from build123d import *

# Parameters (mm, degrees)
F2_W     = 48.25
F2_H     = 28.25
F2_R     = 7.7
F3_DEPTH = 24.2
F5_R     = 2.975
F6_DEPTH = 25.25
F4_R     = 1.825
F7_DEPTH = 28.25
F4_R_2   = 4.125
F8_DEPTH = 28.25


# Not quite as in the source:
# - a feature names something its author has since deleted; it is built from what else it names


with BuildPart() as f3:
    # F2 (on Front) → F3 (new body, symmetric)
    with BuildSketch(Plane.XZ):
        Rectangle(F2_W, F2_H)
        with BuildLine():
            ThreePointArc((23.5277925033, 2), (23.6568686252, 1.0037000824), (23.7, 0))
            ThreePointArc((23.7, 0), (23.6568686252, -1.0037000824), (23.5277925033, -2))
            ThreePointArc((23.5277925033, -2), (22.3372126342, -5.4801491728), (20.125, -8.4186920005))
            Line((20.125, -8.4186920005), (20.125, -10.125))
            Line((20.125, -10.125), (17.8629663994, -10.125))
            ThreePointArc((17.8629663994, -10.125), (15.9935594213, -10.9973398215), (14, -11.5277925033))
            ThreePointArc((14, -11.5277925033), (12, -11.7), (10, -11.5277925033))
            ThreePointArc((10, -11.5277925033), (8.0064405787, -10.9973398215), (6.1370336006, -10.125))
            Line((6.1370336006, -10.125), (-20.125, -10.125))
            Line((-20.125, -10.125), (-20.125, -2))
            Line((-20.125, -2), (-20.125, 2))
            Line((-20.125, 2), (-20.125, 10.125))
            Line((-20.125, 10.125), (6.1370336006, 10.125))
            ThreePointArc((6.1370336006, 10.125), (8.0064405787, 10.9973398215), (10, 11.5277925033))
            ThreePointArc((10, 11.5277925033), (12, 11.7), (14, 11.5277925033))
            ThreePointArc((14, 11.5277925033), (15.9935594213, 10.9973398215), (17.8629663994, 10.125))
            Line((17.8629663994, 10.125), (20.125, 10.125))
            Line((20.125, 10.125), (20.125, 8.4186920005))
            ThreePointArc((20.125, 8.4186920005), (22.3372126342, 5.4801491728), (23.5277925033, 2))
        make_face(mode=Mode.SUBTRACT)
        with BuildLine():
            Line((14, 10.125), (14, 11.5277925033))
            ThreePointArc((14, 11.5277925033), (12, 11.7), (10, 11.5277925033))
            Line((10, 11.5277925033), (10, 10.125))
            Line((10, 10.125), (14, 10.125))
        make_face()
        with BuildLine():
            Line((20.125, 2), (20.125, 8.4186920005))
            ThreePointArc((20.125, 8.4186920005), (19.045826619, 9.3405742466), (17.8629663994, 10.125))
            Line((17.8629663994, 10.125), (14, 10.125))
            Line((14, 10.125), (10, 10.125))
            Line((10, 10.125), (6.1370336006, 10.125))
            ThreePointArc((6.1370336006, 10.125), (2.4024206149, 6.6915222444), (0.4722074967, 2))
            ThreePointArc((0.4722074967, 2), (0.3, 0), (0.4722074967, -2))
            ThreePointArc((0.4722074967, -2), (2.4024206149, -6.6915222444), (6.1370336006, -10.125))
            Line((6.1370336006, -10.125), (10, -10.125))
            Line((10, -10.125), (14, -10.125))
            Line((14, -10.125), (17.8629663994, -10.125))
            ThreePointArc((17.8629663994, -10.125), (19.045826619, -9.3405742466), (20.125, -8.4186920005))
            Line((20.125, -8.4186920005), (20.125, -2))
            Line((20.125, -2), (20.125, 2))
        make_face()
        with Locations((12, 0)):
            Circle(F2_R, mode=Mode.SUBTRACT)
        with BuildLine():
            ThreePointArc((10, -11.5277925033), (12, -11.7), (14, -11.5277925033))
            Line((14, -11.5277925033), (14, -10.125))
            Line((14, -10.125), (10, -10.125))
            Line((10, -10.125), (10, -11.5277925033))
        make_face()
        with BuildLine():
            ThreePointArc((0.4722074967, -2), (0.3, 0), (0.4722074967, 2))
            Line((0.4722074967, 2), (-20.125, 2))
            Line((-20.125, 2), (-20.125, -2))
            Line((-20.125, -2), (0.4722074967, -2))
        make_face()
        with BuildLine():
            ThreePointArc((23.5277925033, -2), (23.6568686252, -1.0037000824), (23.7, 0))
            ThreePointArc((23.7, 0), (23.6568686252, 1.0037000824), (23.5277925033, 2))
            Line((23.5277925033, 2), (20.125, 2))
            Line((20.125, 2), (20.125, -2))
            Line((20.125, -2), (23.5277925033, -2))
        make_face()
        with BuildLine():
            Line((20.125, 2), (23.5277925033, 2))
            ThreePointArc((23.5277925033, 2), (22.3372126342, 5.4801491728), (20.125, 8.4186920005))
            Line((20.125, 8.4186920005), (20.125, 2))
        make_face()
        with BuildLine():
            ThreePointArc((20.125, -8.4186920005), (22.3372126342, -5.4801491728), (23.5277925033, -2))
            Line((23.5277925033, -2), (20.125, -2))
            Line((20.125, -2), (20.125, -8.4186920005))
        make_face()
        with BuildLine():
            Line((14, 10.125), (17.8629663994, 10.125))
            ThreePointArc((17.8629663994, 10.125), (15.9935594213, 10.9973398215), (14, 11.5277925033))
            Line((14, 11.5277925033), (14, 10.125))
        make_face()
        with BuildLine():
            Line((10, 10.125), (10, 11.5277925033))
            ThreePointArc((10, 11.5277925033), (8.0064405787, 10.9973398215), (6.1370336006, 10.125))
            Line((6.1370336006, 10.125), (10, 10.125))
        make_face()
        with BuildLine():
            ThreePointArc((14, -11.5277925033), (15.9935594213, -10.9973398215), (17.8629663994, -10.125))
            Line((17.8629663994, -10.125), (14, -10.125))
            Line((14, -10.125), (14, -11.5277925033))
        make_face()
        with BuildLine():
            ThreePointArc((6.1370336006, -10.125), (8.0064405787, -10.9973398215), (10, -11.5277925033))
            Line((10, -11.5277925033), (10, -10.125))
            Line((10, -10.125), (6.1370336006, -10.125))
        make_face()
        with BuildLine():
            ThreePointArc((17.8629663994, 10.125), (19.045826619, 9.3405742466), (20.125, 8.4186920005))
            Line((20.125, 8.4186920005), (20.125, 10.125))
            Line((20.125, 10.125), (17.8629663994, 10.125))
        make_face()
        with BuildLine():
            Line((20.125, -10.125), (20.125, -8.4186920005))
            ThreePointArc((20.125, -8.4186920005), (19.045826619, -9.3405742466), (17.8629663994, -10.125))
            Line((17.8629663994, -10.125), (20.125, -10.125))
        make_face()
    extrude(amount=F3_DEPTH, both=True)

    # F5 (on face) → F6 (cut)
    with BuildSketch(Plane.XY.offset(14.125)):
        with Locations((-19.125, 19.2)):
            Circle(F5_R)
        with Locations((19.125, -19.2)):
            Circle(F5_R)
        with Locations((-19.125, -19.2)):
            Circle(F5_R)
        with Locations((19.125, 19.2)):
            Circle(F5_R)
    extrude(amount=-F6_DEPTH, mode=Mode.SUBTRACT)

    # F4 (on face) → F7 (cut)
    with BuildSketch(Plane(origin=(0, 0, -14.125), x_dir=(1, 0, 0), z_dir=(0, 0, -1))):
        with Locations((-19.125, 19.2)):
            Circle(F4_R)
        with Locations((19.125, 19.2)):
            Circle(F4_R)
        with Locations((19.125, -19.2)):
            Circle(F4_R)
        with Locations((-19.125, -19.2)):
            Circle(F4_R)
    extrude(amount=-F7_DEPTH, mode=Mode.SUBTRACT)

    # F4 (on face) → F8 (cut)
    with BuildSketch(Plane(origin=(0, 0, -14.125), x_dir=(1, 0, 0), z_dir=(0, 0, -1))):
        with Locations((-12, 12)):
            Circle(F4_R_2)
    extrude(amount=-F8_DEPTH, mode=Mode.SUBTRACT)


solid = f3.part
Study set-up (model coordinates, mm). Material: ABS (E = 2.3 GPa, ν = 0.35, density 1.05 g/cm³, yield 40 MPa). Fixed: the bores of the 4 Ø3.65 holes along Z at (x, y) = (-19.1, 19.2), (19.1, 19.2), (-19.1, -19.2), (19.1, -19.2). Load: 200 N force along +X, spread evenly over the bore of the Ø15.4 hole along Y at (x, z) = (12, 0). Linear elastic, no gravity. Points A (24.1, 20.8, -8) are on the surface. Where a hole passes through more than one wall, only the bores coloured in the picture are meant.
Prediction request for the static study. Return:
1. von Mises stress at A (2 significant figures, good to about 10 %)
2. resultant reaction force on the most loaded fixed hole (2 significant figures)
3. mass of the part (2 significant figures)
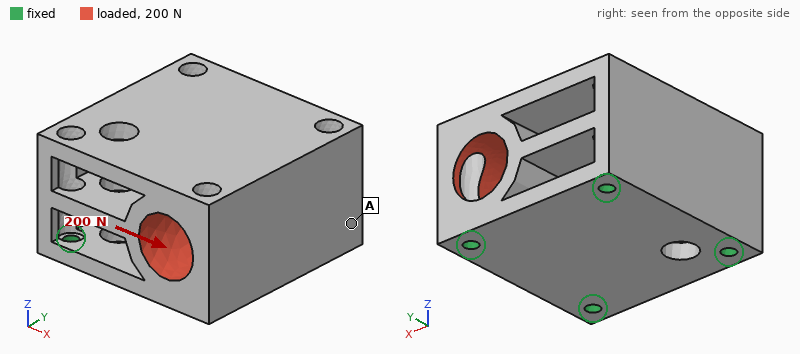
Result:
0.69 MPa
73 N
38 g
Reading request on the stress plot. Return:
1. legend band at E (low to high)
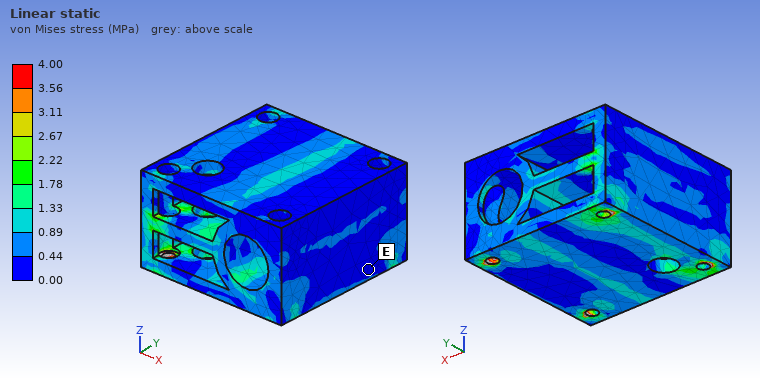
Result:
0.00 to 0.44 MPa
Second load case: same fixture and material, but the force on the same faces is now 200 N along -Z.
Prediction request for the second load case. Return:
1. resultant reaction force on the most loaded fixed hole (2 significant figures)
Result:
86 N
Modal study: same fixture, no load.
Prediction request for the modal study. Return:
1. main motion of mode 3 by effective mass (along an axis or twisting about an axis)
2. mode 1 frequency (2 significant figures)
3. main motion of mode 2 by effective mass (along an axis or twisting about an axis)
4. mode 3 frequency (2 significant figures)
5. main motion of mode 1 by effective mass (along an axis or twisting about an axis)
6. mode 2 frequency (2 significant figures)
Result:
along Z
1600 Hz
along Y
3200 Hz
along X
2900 Hz
